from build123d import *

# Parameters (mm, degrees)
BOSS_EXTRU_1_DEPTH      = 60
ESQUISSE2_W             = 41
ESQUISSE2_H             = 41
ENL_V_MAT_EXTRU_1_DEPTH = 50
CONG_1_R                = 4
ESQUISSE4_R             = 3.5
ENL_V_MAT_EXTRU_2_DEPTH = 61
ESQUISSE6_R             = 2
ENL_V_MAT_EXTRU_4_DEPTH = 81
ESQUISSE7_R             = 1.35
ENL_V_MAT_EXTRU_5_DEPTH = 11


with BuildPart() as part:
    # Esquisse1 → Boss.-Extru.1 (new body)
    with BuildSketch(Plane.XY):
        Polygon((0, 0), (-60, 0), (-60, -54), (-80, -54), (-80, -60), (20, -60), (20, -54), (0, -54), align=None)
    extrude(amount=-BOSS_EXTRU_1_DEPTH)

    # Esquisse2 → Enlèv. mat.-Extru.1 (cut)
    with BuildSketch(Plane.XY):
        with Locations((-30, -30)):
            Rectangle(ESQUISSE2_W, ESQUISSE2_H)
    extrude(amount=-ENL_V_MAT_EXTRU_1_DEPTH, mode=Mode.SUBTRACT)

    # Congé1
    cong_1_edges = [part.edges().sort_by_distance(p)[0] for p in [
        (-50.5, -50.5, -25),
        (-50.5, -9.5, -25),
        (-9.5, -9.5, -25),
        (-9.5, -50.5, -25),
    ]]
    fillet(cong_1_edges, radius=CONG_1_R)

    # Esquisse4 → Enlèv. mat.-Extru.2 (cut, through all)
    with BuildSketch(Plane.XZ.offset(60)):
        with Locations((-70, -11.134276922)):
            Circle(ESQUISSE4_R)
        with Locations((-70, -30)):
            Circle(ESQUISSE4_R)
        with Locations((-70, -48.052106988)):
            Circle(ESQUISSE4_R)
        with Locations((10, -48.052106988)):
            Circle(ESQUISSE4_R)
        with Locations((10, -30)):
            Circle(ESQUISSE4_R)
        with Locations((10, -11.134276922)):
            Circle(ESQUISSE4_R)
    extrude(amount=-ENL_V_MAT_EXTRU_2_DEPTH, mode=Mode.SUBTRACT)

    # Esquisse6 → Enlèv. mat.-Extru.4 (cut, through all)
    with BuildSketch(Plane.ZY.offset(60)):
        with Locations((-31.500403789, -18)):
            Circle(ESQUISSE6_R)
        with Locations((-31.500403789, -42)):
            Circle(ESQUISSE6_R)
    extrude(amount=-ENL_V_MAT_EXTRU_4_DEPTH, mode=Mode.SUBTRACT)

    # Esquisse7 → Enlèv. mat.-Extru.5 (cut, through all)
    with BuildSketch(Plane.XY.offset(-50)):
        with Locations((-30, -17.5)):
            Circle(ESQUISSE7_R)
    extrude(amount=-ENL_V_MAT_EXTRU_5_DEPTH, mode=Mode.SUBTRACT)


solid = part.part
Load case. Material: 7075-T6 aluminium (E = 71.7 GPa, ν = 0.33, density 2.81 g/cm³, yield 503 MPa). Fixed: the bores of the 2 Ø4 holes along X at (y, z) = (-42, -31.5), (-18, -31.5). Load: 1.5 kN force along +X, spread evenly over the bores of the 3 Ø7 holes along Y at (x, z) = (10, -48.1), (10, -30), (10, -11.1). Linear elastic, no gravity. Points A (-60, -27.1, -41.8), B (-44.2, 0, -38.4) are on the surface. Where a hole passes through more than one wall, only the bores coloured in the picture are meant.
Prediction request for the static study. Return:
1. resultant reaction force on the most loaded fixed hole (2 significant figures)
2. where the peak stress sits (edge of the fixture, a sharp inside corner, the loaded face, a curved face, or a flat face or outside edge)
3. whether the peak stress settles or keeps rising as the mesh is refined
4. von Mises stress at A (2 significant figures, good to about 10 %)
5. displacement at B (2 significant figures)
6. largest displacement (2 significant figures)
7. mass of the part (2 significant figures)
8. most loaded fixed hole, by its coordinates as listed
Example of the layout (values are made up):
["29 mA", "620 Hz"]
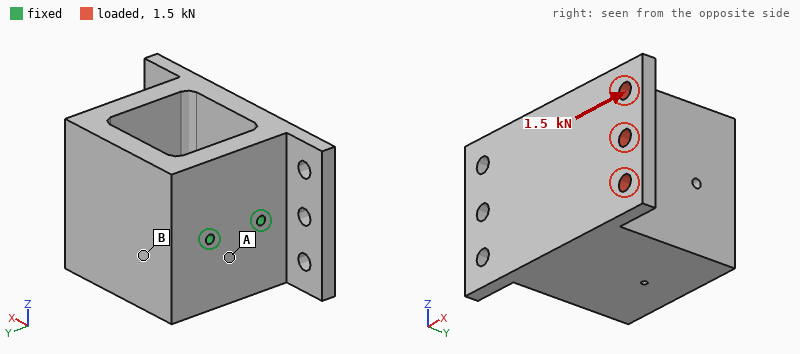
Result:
["2.0 kN", "edge of the fixture", "keeps rising", "4.7 MPa", "6.7 µm", "30 µm", "410 g", "(-42, -31.5)"]
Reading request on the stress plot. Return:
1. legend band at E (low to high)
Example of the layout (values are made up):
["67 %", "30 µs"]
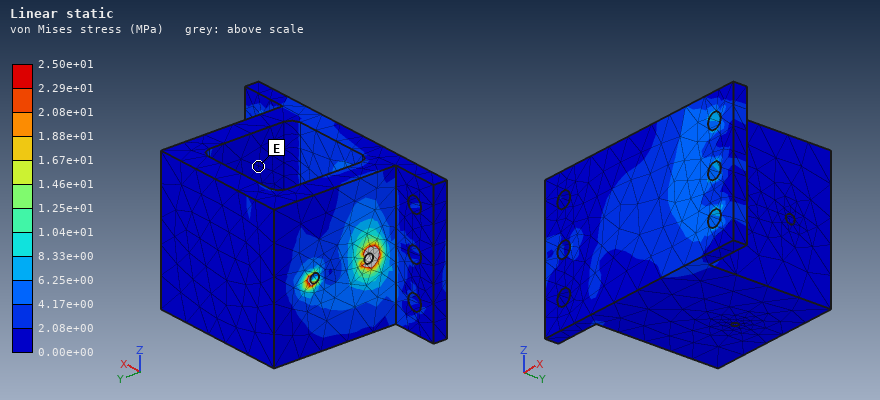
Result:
["0.00e+00 to 2.08e+00 MPa"]
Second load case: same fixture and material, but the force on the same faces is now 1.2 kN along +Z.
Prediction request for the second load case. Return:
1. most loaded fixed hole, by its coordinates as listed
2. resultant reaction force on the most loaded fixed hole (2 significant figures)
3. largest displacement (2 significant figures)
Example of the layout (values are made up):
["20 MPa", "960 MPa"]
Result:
["(-42, -31.5)", "1.8 kN", "0.19 mm"]
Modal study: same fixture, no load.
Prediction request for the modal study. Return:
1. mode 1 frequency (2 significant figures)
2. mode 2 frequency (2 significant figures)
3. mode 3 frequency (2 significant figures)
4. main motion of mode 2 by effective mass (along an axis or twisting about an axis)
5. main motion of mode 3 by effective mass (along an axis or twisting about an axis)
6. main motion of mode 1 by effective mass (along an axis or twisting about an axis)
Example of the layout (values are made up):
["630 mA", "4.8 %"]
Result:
["1200 Hz", "1900 Hz", "4100 Hz", "along Y", "twisting about X", "along Z"]
